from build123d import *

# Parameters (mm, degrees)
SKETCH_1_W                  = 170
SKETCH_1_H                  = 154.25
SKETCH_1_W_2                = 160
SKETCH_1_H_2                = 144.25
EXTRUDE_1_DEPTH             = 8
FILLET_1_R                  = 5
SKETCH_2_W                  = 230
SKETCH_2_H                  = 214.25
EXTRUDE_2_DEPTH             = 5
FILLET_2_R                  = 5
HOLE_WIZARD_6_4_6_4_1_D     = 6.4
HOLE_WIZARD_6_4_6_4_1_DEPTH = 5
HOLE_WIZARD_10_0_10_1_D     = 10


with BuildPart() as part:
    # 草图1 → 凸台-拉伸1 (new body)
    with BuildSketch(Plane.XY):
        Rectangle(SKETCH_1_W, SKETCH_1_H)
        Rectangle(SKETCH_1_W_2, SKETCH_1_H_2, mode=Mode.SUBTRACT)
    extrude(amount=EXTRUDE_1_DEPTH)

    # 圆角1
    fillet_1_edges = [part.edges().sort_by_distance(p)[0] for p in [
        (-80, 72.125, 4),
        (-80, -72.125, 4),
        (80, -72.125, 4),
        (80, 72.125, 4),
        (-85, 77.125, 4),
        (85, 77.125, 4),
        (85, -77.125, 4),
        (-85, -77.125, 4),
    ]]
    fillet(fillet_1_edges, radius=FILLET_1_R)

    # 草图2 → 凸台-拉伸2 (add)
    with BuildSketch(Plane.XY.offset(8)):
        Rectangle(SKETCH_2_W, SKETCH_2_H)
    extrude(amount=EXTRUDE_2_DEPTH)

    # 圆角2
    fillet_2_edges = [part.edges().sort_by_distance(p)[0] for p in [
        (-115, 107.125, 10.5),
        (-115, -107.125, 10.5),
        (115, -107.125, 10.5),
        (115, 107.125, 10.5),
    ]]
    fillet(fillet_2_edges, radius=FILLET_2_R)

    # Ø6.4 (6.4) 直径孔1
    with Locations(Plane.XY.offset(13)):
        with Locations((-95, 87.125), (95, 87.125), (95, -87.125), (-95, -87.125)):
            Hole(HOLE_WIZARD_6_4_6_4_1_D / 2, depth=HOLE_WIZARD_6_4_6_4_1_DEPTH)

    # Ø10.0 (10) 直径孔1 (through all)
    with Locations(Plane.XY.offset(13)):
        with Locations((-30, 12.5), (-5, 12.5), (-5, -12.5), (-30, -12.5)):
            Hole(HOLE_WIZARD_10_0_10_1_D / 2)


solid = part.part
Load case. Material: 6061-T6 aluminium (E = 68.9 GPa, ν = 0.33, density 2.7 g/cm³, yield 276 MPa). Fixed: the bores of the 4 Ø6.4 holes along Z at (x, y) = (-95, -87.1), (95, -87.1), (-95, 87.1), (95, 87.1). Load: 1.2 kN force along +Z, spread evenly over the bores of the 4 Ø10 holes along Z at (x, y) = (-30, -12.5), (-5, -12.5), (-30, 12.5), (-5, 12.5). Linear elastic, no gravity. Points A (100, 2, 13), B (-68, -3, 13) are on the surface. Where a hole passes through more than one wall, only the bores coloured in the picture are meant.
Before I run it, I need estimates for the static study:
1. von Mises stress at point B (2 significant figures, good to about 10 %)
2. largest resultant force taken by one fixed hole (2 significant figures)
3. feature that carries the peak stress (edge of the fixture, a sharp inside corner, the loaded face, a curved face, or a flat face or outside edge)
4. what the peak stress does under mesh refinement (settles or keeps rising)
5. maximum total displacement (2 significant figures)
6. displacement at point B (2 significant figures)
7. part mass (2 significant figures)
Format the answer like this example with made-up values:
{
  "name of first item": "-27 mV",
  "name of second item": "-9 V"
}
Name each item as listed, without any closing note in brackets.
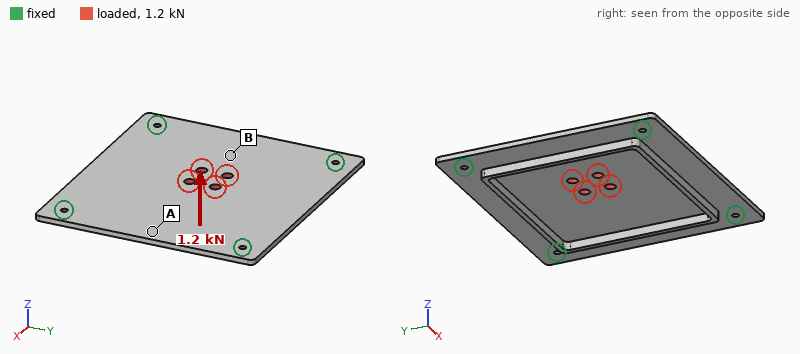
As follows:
{
  "von Mises stress at point B": "20 MPa",
  "largest resultant force taken by one fixed hole": "610 N",
  "feature that carries the peak stress": "edge of the fixture",
  "what the peak stress does under mesh refinement": "keeps rising",
  "maximum total displacement": "0.56 mm",
  "displacement at point B": "0.29 mm",
  "part mass": "730 g"
}
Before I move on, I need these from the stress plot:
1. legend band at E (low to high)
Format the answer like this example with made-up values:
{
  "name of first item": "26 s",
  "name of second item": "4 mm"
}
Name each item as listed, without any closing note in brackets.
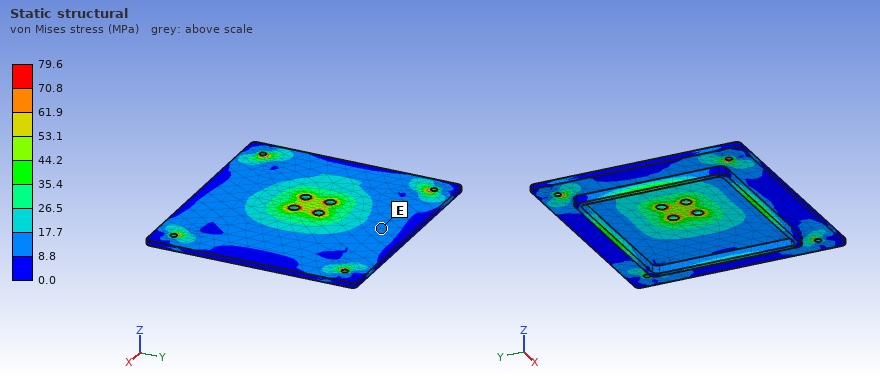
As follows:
{
  "legend band at E": "8.8 to 17.7 MPa"
}
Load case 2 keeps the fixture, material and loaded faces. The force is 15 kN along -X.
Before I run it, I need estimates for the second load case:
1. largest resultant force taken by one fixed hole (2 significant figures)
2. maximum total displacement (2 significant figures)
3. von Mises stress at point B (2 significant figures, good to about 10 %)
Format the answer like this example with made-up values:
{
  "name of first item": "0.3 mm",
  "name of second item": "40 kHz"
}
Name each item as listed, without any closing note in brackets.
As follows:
{
  "largest resultant force taken by one fixed hole": "4.2 kN",
  "maximum total displacement": "43 µm",
  "von Mises stress at point B": "9.1 MPa"
}
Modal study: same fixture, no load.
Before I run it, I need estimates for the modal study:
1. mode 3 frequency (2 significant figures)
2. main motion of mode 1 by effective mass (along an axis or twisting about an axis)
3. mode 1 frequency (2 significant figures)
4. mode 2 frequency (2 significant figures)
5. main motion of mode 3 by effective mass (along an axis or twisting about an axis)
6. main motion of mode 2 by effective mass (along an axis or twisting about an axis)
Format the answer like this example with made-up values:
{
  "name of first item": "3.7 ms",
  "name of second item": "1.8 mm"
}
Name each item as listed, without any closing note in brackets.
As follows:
{
  "mode 3 frequency": "1100 Hz",
  "main motion of mode 1 by effective mass": "along Z",
  "mode 1 frequency": "610 Hz",
  "mode 2 frequency": "960 Hz",
  "main motion of mode 3 by effective mass": "twisting about Y",
  "main motion of mode 2 by effective mass": "twisting about X"
}
